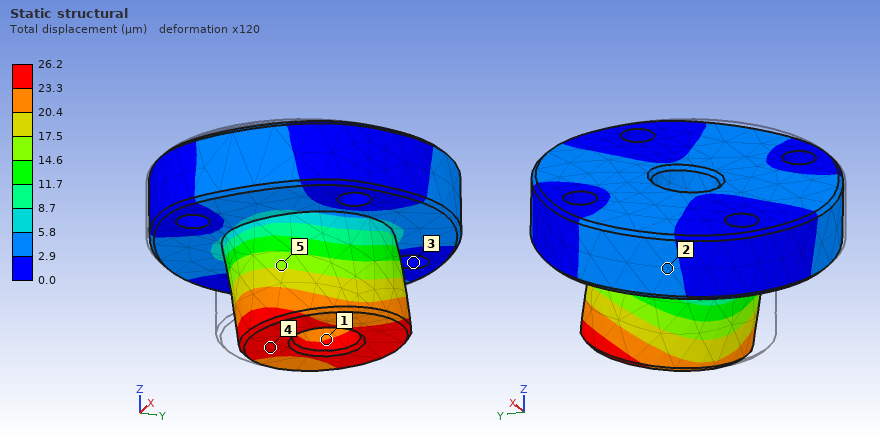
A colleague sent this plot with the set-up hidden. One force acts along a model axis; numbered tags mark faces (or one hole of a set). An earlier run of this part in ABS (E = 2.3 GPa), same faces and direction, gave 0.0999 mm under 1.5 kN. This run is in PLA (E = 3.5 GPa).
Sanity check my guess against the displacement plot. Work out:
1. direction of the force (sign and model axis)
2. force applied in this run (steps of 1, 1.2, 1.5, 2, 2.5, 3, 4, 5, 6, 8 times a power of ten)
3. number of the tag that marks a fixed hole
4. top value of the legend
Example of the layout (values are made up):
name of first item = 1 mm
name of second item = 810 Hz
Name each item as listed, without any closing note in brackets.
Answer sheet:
direction of the force = +Y
force applied in this run = 600 N
number of the tag that marks a fixed hole = 3
top value of the legend = 26.2 µm
